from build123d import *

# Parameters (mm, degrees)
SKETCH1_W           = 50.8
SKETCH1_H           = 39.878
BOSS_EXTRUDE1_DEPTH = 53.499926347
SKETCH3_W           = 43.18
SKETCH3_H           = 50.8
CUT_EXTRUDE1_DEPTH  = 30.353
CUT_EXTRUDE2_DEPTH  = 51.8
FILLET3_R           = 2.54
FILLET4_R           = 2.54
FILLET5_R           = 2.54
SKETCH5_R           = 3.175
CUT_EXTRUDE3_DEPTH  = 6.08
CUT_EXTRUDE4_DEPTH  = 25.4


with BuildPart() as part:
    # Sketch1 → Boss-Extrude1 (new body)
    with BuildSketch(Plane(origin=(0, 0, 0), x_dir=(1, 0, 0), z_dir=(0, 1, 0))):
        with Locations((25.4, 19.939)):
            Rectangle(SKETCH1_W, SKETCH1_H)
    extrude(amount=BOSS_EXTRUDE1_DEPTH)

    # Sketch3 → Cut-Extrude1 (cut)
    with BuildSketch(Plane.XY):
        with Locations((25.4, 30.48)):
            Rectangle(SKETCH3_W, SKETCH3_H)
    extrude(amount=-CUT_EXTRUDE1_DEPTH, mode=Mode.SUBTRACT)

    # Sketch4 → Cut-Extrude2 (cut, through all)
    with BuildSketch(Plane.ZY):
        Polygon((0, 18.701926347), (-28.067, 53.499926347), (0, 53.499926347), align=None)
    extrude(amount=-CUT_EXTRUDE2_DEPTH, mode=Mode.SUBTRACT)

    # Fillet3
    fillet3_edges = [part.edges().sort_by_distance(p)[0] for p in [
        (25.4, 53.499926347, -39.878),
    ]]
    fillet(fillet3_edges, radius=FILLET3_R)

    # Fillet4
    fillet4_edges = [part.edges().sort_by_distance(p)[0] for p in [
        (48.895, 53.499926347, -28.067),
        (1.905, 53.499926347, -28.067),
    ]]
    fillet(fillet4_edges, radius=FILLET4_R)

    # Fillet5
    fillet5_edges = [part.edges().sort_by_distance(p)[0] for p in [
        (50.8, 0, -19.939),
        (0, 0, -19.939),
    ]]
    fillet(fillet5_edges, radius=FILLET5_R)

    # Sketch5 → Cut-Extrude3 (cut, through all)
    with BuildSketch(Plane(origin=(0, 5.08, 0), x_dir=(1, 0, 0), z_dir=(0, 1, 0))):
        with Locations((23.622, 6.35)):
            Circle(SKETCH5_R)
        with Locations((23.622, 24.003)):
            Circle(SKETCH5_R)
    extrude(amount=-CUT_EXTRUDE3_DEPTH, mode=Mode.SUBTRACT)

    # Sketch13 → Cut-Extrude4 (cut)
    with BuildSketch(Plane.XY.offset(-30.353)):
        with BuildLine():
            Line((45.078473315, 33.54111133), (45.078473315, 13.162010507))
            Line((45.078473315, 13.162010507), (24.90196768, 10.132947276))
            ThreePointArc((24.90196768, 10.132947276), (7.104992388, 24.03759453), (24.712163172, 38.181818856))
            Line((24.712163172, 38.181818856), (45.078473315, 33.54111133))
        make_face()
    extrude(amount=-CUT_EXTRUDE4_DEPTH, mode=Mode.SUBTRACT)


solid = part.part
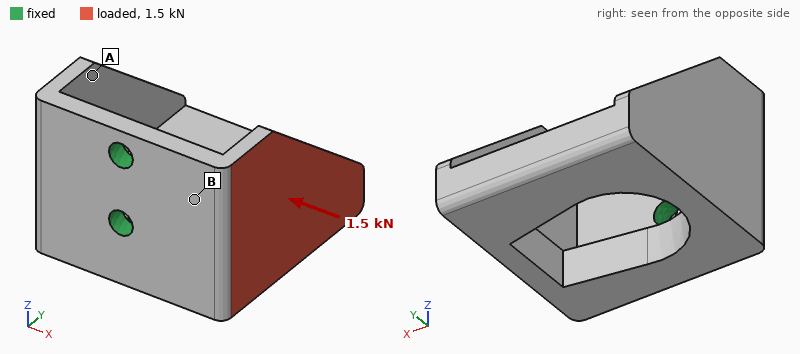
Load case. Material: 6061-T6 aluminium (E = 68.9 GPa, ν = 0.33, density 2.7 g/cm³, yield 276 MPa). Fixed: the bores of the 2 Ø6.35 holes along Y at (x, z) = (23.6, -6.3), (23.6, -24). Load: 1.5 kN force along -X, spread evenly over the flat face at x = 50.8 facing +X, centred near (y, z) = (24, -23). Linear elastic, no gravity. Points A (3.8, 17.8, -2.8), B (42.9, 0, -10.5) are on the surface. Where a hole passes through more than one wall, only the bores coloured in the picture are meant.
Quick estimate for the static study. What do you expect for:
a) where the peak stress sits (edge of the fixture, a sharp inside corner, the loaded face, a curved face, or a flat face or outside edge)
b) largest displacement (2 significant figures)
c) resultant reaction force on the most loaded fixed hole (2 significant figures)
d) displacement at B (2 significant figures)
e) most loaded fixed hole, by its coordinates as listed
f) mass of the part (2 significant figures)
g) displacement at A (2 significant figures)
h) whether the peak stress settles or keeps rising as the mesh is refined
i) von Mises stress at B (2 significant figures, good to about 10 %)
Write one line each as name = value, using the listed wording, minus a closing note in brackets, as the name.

where the peak stress sits = edge of the fixture
largest displacement = 0.30 mm
resultant reaction force on the most loaded fixed hole = 1.2 kN
displacement at B = 0.057 mm
most loaded fixed hole, by its coordinates as listed = (23.6, -24)
mass of the part = 86 g
displacement at A = 0.084 mm
whether the peak stress settles or keeps rising as the mesh is refined = keeps rising
von Mises stress at B = 35 MPa
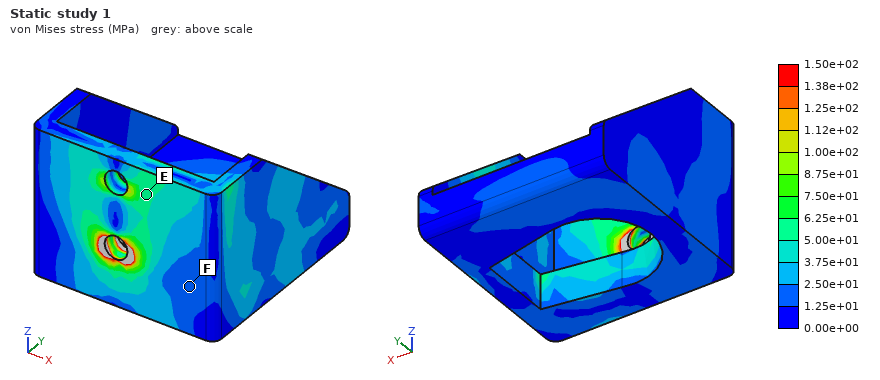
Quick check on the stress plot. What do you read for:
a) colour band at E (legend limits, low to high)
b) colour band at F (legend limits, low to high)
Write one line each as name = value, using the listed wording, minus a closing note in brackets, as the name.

colour band at E = 5.00e+01 to 6.25e+01 MPa
colour band at F = 1.25e+01 to 2.50e+01 MPa
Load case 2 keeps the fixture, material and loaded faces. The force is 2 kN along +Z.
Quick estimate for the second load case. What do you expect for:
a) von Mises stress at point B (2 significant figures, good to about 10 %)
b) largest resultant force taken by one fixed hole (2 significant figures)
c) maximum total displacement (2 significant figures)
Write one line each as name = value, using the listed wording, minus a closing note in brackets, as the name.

von Mises stress at point B = 55 MPa
largest resultant force taken by one fixed hole = 3.1 kN
maximum total displacement = 0.38 mm
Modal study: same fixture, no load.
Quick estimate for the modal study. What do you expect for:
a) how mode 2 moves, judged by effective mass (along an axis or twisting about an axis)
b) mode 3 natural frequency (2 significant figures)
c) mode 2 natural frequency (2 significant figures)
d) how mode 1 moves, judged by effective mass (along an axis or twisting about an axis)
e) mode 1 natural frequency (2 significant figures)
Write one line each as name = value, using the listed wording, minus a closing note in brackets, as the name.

how mode 2 moves, judged by effective mass = along Z
mode 3 natural frequency = 4000 Hz
mode 2 natural frequency = 1900 Hz
how mode 1 moves, judged by effective mass = along X
mode 1 natural frequency = 1500 Hz
